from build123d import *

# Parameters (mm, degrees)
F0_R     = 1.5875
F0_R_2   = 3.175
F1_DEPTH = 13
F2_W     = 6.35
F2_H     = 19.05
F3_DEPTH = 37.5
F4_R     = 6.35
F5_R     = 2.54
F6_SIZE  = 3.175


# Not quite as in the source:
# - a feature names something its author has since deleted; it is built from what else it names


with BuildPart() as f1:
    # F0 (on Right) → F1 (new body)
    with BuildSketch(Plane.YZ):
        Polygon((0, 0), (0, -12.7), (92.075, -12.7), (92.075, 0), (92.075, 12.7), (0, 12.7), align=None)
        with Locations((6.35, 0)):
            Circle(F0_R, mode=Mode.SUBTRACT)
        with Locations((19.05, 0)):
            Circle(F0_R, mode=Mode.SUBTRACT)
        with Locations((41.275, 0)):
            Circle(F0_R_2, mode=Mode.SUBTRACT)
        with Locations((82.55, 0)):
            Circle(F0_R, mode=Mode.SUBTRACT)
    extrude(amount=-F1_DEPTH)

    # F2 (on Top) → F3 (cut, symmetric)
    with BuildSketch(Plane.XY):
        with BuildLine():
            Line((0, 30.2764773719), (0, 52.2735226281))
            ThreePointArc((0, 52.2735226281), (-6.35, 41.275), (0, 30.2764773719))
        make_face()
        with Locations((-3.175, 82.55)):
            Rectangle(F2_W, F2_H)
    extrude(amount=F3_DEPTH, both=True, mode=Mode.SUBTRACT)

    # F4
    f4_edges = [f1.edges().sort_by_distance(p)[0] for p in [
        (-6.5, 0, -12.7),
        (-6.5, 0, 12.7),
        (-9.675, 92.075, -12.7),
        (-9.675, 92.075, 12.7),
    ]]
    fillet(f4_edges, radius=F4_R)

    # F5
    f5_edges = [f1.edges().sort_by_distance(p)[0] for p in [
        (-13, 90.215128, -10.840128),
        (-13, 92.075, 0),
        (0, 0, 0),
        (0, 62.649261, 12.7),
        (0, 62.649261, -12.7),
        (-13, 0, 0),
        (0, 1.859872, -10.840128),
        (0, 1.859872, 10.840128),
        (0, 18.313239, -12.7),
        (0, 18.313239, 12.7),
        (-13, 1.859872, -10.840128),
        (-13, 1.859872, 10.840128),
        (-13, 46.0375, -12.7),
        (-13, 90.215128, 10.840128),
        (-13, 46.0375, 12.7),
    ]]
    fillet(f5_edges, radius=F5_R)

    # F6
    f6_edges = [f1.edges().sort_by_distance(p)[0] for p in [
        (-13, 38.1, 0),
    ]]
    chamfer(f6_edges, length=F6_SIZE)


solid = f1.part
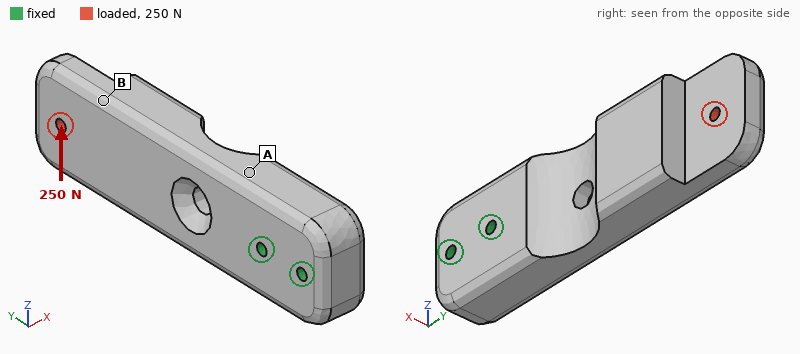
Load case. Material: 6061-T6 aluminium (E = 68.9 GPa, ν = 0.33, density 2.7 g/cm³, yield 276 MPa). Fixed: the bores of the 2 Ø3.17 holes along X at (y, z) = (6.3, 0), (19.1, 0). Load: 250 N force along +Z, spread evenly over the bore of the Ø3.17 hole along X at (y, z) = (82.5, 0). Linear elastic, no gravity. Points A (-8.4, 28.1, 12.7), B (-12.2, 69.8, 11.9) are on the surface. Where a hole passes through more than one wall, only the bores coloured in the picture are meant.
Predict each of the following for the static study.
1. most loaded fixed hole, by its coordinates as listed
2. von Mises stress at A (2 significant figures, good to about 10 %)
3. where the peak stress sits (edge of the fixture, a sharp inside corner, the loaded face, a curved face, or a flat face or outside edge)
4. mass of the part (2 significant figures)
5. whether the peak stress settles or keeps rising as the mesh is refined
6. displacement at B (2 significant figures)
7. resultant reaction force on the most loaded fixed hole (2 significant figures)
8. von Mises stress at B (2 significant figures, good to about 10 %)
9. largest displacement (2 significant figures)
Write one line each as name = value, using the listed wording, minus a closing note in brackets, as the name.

most loaded fixed hole, by its coordinates as listed = (19.1, 0)
von Mises stress at A = 14 MPa
where the peak stress sits = edge of the fixture
mass of the part = 63 g
whether the peak stress settles or keeps rising as the mesh is refined = keeps rising
displacement at B = 35 µm
resultant reaction force on the most loaded fixed hole = 1.2 kN
von Mises stress at B = 4.1 MPa
largest displacement = 53 µm
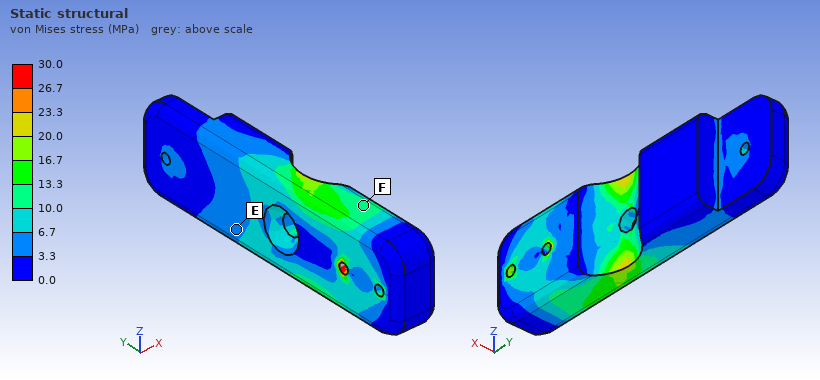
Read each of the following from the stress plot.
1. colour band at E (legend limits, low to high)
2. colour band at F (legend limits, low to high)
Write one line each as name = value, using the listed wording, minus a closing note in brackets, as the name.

colour band at E = 3.3 to 6.7 MPa
colour band at F = 10.0 to 13.3 MPa
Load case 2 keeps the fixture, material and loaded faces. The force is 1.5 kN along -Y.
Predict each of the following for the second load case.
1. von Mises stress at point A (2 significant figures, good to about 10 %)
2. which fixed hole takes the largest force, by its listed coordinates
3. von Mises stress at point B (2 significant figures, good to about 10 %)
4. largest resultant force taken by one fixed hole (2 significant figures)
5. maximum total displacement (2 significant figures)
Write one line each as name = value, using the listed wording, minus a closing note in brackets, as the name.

von Mises stress at point A = 6.6 MPa
which fixed hole takes the largest force, by its listed coordinates = (19.1, 0)
von Mises stress at point B = 9.3 MPa
largest resultant force taken by one fixed hole = 1.1 kN
maximum total displacement = 48 µm
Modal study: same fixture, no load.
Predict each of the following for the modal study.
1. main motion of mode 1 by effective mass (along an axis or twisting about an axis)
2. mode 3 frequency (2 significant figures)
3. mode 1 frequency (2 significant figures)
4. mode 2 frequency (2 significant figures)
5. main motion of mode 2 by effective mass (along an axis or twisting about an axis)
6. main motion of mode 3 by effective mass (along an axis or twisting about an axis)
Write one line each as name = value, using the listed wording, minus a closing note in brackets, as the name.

main motion of mode 1 by effective mass = along X
mode 3 frequency = 6500 Hz
mode 1 frequency = 1300 Hz
mode 2 frequency = 2900 Hz
main motion of mode 2 by effective mass = along Z
main motion of mode 3 by effective mass = twisting about Y
